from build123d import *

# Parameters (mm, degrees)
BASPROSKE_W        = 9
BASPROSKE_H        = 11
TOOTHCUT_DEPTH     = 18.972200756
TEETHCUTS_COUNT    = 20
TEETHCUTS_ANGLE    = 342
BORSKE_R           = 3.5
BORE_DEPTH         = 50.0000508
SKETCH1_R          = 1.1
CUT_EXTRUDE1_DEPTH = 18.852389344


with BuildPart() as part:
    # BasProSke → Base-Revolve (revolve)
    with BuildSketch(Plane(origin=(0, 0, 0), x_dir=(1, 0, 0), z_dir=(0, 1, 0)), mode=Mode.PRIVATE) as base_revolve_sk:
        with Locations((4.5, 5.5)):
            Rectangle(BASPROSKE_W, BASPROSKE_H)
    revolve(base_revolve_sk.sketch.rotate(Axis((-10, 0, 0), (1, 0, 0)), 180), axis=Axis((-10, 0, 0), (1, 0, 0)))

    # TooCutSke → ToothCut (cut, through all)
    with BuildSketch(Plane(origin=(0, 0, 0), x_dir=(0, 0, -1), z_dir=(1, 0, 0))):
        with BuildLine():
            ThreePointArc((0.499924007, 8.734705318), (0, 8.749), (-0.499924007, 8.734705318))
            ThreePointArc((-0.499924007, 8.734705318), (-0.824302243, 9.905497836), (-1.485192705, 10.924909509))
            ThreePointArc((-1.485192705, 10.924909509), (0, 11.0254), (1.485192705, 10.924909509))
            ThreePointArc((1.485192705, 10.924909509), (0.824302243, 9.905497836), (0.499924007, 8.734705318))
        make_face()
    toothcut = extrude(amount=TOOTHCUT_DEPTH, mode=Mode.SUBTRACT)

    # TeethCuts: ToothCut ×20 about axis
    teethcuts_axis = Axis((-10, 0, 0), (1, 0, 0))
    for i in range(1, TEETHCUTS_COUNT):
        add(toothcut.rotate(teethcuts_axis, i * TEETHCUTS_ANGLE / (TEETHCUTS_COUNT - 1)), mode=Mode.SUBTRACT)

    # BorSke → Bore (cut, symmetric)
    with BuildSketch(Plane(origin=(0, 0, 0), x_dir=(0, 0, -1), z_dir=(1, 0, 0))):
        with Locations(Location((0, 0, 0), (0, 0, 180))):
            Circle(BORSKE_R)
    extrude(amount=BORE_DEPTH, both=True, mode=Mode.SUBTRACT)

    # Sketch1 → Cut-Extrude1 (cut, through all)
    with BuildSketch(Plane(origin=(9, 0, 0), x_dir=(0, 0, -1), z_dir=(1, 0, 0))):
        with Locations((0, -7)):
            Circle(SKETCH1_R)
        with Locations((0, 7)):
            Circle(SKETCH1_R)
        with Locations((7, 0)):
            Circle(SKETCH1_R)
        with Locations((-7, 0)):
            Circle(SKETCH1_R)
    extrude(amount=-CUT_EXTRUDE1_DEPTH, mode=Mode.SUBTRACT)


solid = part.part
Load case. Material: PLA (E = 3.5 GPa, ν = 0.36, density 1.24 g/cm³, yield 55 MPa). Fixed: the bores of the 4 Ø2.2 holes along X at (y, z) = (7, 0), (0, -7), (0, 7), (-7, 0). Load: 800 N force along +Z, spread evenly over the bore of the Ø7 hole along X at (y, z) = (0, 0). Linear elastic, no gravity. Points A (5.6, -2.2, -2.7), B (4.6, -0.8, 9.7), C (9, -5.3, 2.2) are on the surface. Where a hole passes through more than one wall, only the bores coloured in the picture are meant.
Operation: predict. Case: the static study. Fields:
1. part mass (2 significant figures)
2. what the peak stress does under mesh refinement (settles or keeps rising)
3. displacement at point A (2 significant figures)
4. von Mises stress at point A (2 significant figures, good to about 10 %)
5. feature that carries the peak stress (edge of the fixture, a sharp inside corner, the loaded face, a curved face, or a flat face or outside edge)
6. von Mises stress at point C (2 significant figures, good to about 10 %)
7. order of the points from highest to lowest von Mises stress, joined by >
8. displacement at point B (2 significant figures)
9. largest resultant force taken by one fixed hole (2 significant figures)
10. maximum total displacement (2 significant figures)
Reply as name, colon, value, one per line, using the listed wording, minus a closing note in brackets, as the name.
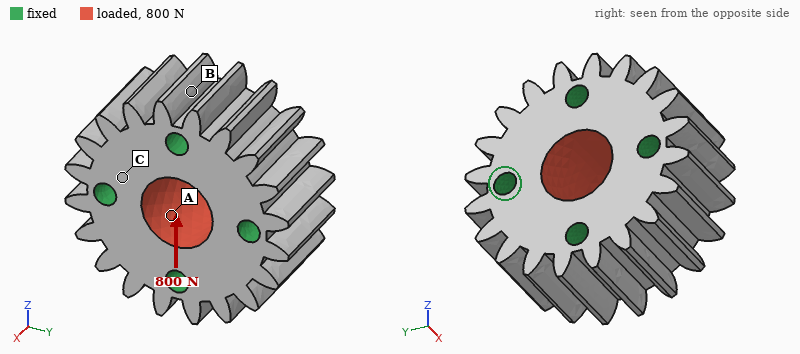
part mass: 2.8 g
what the peak stress does under mesh refinement: keeps rising
displacement at point A: 6.7 µm
von Mises stress at point A: 5.1 MPa
feature that carries the peak stress: edge of the fixture
von Mises stress at point C: 2.8 MPa
order of the points from highest to lowest von Mises stress, joined by >: A > C > B
displacement at point B: 1.4 µm
largest resultant force taken by one fixed hole: 230 N
maximum total displacement: 8.0 µm
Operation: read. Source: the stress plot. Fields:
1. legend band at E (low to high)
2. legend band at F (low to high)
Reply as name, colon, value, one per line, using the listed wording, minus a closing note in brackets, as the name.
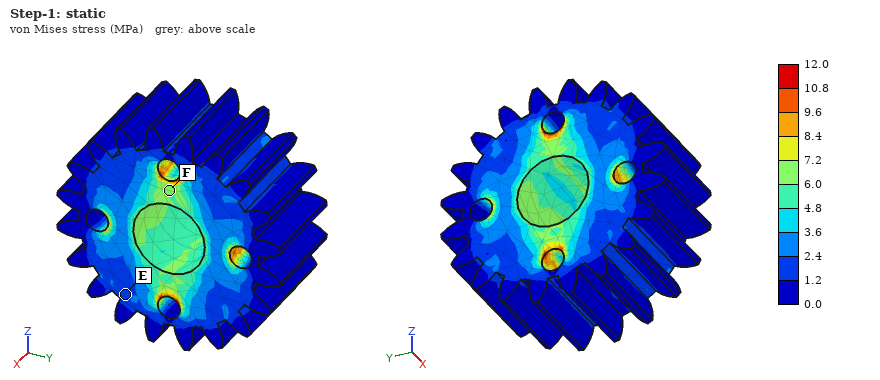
legend band at E: 1.2 to 2.4 MPa
legend band at F: 6.0 to 7.2 MPa
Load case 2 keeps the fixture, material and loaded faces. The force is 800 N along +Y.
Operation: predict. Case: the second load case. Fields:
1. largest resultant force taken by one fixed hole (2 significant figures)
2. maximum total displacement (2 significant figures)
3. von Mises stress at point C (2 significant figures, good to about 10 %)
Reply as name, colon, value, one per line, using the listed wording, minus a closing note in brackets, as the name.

largest resultant force taken by one fixed hole: 230 N
maximum total displacement: 8.0 µm
von Mises stress at point C: 3.8 MPa
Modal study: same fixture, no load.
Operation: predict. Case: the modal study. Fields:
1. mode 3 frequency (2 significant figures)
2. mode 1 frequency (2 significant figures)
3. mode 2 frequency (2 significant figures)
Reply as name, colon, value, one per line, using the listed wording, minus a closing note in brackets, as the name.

mode 3 frequency: 36 kHz
mode 1 frequency: 34 kHz
mode 2 frequency: 36 kHz
